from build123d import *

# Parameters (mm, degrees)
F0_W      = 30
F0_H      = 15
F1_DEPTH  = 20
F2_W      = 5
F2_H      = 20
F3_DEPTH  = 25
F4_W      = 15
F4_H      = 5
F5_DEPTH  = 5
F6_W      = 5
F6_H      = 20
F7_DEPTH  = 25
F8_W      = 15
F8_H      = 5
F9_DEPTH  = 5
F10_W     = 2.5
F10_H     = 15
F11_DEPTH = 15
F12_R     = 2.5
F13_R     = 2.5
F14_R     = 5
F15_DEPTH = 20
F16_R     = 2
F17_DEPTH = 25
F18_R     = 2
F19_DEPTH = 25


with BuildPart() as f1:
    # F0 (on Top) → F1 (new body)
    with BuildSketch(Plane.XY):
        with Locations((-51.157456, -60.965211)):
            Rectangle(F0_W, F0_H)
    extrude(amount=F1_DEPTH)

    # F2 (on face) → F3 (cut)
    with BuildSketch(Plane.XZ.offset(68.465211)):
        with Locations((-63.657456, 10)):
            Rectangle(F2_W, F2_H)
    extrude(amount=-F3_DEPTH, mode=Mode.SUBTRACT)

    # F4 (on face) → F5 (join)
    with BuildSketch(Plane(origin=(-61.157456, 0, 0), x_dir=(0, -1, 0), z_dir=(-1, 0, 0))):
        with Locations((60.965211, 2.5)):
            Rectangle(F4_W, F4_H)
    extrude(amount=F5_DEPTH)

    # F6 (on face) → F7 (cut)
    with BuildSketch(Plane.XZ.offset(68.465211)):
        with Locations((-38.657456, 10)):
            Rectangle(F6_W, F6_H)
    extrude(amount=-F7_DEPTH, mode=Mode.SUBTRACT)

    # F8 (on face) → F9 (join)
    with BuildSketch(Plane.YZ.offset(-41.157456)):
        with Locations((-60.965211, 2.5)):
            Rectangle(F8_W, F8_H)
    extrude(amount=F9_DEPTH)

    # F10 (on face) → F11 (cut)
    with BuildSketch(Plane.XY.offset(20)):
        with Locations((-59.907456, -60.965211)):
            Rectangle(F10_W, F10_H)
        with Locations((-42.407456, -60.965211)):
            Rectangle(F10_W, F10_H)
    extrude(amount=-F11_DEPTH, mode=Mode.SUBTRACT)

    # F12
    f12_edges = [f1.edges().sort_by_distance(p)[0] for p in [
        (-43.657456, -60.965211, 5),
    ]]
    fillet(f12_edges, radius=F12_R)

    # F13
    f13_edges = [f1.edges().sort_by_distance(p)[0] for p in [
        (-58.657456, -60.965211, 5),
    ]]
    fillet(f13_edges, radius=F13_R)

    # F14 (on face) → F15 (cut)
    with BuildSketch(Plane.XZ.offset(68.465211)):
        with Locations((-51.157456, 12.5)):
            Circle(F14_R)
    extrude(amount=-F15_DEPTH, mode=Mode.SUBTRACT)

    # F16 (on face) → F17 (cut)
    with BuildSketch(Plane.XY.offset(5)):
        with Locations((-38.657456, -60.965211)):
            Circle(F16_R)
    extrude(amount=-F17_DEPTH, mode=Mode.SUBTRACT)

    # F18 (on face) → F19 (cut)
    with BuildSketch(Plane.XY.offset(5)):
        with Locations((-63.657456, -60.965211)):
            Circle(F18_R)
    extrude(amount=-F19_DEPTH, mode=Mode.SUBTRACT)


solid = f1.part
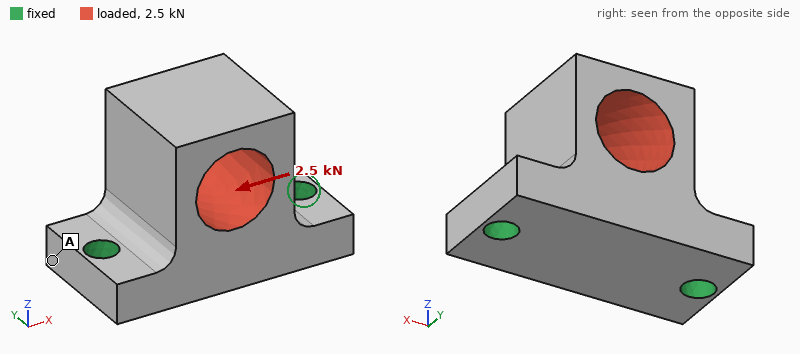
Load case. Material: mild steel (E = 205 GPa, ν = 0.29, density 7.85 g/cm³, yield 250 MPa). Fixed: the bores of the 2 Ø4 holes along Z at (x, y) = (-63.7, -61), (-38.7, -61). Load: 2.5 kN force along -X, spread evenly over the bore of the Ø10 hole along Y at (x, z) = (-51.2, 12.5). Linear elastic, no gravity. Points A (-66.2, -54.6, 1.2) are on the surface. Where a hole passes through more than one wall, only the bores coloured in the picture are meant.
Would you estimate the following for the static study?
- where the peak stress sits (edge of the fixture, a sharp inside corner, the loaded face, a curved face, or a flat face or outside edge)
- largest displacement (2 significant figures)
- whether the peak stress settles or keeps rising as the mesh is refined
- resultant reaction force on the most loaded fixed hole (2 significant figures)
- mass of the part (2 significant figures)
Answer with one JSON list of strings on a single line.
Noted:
["edge of the fixture", "14 µm", "keeps rising", "1.7 kN", "34 g"]
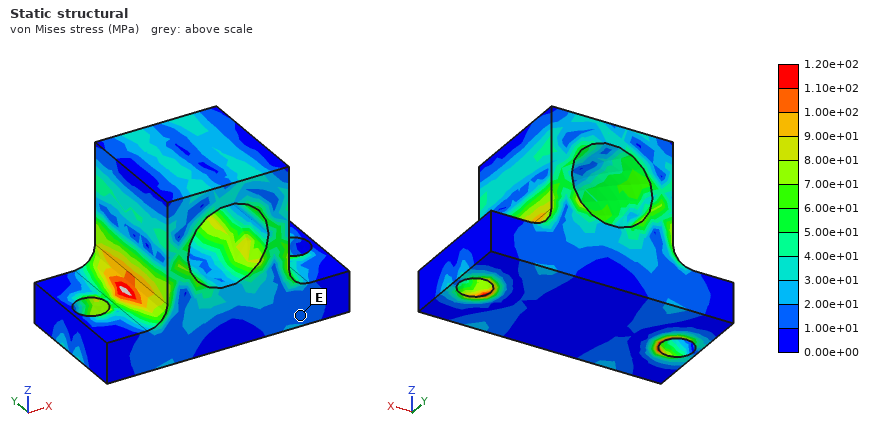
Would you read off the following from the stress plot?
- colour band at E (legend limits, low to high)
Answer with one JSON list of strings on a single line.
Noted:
["1.00e+01 to 2.00e+01 MPa"]
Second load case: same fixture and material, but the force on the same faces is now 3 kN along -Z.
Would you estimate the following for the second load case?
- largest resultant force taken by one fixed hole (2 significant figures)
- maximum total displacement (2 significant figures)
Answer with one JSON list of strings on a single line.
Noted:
["1.6 kN", "5.1 µm"]
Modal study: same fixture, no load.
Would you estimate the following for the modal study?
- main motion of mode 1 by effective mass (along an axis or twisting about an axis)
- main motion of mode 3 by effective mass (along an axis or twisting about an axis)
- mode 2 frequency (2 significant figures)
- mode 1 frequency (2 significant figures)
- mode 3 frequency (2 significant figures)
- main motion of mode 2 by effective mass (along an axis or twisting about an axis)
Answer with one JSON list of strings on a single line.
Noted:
["along Y", "along Z", "18 kHz", "12 kHz", "28 kHz", "along X"]
